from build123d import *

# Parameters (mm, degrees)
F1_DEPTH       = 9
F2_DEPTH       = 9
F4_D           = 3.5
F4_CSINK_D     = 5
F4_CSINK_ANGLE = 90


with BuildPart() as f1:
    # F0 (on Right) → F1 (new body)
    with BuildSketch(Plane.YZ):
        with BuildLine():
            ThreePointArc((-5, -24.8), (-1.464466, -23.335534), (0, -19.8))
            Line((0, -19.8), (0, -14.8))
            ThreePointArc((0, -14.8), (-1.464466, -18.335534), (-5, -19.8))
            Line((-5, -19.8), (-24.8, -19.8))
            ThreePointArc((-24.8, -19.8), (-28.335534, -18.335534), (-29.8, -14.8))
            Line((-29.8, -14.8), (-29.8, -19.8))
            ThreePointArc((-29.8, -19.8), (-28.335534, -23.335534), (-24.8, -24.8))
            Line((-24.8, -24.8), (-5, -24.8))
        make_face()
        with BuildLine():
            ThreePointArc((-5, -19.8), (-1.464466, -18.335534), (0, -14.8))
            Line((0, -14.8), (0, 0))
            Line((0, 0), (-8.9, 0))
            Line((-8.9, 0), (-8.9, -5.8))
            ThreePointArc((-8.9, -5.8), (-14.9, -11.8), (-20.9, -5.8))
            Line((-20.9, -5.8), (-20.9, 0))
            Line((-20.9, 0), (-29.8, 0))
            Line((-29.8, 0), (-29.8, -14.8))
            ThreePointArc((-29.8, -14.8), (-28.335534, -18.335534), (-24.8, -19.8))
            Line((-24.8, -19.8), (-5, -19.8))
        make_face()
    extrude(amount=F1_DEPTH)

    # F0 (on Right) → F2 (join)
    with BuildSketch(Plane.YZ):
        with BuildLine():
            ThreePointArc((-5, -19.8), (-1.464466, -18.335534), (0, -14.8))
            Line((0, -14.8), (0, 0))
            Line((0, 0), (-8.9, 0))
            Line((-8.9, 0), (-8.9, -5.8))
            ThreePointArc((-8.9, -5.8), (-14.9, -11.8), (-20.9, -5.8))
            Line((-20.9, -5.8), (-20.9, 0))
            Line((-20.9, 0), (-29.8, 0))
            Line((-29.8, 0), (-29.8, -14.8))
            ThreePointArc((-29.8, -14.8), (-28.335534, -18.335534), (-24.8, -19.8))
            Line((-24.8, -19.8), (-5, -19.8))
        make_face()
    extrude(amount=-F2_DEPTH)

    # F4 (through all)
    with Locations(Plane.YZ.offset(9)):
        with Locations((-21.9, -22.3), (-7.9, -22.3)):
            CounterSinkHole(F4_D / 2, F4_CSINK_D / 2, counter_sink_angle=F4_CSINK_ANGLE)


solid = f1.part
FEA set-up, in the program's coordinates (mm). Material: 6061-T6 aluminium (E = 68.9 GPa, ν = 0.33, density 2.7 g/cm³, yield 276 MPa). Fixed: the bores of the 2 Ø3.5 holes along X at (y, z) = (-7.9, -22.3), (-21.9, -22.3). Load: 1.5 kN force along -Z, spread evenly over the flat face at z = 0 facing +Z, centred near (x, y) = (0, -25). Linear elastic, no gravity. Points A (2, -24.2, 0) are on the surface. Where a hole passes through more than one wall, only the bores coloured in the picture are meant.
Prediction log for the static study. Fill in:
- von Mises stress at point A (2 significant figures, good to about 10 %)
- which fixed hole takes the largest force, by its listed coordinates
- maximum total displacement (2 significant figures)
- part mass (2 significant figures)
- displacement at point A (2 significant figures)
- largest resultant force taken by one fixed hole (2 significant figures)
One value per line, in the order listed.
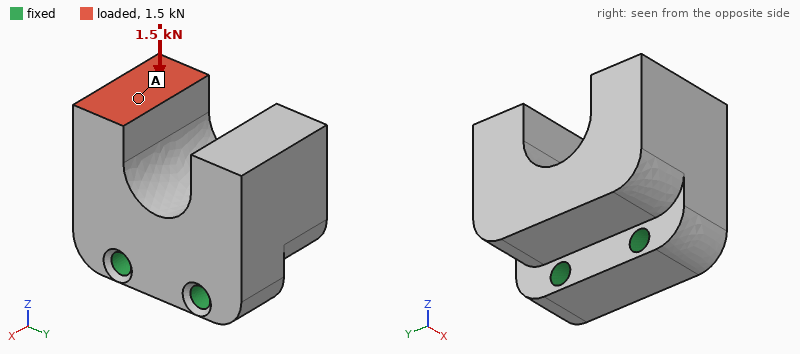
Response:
9.7 MPa
(-21.9, -22.3)
22 µm
25 g
16 µm
1.7 kN
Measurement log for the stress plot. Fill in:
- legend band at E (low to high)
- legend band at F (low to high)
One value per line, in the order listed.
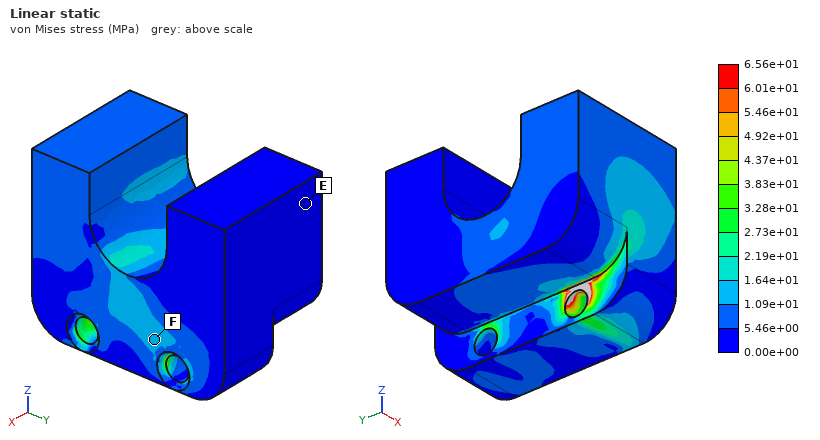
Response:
0.00e+00 to 5.46e+00 MPa
1.09e+01 to 1.64e+01 MPa
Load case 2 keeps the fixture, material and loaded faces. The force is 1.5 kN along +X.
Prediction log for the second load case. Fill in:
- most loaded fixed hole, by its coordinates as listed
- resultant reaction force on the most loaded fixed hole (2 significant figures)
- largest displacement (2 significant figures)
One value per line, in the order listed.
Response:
(-21.9, -22.3)
1.4 kN
86 µm
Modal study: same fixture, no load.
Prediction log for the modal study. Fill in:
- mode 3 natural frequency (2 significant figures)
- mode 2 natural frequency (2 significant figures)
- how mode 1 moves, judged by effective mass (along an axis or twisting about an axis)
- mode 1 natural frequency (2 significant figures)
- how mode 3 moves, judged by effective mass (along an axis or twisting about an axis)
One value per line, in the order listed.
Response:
16 kHz
15 kHz
along X
9600 Hz
along Y
